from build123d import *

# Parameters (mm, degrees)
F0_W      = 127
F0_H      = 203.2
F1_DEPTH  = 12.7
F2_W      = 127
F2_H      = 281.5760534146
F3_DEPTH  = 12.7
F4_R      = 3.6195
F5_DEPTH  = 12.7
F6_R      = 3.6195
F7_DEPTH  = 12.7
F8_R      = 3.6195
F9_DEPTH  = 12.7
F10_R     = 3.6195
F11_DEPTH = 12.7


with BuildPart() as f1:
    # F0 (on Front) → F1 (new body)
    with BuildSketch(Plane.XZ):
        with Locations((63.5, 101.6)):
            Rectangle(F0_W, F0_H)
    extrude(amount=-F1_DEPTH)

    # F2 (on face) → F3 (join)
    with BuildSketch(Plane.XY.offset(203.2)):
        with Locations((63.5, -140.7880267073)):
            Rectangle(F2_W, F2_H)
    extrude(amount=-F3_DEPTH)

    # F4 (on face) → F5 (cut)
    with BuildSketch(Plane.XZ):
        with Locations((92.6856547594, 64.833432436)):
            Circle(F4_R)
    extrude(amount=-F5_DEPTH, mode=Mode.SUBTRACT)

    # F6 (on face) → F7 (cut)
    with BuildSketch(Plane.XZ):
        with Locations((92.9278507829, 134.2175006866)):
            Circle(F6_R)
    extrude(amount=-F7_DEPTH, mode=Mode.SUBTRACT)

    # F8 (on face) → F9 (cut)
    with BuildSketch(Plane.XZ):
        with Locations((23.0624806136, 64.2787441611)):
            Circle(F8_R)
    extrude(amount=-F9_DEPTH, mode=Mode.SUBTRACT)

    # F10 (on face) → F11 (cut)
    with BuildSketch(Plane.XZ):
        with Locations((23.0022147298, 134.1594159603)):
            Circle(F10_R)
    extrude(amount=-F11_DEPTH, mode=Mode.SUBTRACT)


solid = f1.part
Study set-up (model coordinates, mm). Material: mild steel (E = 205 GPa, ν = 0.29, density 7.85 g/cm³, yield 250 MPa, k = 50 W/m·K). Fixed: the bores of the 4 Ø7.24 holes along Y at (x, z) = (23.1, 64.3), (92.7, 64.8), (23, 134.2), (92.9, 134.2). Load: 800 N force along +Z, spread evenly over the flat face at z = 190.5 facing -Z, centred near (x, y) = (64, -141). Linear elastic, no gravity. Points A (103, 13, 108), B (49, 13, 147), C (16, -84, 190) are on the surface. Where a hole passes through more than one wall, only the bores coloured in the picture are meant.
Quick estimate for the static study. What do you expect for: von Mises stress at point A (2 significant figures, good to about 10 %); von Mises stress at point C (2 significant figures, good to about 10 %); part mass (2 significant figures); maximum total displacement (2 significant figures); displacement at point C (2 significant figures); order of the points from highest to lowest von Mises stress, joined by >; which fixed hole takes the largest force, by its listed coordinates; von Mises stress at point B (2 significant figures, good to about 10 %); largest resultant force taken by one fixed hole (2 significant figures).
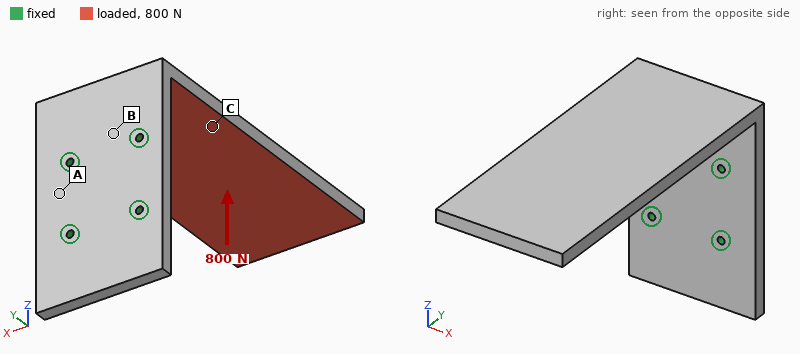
6.3 MPa
16 MPa
6.1 kg
0.98 mm
0.22 mm
B > C > A
(92.9, 134.2)
26 MPa
580 N
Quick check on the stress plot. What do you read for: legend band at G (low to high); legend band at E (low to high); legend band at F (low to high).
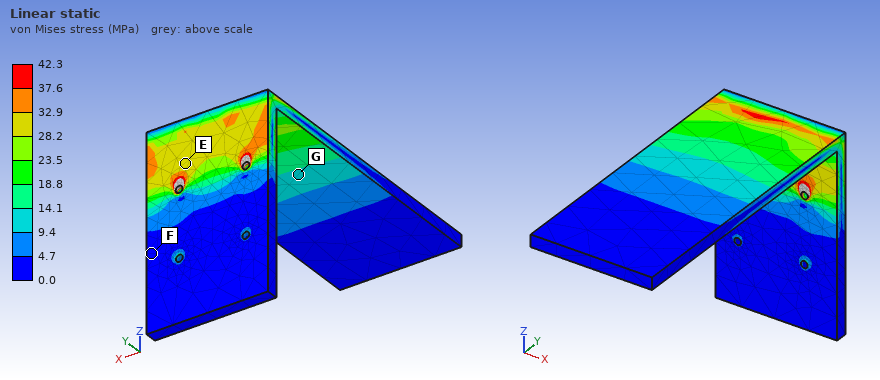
9.4 to 14.1 MPa
28.2 to 32.9 MPa
0.0 to 4.7 MPa
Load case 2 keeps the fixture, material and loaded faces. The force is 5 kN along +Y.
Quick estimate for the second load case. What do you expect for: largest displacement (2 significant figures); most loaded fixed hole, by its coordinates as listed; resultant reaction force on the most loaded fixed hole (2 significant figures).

0.41 mm
(92.9, 134.2)
3.7 kN
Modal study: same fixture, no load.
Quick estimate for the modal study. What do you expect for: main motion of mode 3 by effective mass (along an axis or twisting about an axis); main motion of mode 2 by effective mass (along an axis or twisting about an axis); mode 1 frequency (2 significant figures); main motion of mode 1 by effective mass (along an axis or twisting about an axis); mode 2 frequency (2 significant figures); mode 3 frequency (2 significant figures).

along Y
along X
94 Hz
along Z
230 Hz
550 Hz
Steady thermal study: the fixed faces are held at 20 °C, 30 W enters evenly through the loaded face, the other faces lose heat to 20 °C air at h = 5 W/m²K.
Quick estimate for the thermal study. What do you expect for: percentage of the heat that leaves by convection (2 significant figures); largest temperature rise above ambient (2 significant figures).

35 %
52 K
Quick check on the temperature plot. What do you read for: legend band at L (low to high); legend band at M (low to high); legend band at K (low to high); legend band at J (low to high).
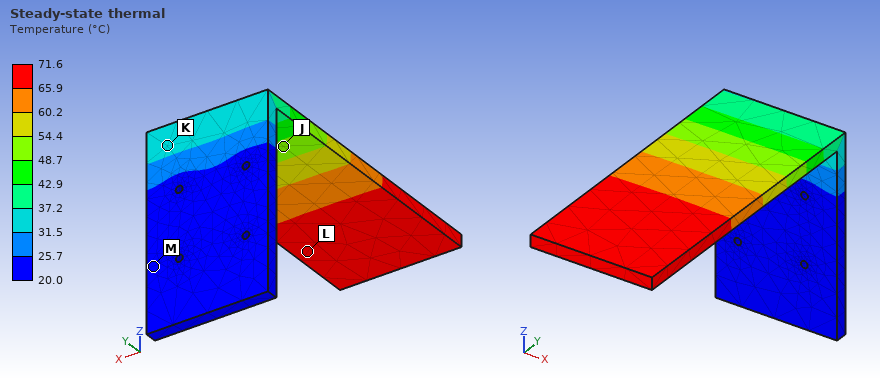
65.9 to 71.6 °C
20.0 to 25.7 °C
31.5 to 37.2 °C
48.7 to 54.4 °C
